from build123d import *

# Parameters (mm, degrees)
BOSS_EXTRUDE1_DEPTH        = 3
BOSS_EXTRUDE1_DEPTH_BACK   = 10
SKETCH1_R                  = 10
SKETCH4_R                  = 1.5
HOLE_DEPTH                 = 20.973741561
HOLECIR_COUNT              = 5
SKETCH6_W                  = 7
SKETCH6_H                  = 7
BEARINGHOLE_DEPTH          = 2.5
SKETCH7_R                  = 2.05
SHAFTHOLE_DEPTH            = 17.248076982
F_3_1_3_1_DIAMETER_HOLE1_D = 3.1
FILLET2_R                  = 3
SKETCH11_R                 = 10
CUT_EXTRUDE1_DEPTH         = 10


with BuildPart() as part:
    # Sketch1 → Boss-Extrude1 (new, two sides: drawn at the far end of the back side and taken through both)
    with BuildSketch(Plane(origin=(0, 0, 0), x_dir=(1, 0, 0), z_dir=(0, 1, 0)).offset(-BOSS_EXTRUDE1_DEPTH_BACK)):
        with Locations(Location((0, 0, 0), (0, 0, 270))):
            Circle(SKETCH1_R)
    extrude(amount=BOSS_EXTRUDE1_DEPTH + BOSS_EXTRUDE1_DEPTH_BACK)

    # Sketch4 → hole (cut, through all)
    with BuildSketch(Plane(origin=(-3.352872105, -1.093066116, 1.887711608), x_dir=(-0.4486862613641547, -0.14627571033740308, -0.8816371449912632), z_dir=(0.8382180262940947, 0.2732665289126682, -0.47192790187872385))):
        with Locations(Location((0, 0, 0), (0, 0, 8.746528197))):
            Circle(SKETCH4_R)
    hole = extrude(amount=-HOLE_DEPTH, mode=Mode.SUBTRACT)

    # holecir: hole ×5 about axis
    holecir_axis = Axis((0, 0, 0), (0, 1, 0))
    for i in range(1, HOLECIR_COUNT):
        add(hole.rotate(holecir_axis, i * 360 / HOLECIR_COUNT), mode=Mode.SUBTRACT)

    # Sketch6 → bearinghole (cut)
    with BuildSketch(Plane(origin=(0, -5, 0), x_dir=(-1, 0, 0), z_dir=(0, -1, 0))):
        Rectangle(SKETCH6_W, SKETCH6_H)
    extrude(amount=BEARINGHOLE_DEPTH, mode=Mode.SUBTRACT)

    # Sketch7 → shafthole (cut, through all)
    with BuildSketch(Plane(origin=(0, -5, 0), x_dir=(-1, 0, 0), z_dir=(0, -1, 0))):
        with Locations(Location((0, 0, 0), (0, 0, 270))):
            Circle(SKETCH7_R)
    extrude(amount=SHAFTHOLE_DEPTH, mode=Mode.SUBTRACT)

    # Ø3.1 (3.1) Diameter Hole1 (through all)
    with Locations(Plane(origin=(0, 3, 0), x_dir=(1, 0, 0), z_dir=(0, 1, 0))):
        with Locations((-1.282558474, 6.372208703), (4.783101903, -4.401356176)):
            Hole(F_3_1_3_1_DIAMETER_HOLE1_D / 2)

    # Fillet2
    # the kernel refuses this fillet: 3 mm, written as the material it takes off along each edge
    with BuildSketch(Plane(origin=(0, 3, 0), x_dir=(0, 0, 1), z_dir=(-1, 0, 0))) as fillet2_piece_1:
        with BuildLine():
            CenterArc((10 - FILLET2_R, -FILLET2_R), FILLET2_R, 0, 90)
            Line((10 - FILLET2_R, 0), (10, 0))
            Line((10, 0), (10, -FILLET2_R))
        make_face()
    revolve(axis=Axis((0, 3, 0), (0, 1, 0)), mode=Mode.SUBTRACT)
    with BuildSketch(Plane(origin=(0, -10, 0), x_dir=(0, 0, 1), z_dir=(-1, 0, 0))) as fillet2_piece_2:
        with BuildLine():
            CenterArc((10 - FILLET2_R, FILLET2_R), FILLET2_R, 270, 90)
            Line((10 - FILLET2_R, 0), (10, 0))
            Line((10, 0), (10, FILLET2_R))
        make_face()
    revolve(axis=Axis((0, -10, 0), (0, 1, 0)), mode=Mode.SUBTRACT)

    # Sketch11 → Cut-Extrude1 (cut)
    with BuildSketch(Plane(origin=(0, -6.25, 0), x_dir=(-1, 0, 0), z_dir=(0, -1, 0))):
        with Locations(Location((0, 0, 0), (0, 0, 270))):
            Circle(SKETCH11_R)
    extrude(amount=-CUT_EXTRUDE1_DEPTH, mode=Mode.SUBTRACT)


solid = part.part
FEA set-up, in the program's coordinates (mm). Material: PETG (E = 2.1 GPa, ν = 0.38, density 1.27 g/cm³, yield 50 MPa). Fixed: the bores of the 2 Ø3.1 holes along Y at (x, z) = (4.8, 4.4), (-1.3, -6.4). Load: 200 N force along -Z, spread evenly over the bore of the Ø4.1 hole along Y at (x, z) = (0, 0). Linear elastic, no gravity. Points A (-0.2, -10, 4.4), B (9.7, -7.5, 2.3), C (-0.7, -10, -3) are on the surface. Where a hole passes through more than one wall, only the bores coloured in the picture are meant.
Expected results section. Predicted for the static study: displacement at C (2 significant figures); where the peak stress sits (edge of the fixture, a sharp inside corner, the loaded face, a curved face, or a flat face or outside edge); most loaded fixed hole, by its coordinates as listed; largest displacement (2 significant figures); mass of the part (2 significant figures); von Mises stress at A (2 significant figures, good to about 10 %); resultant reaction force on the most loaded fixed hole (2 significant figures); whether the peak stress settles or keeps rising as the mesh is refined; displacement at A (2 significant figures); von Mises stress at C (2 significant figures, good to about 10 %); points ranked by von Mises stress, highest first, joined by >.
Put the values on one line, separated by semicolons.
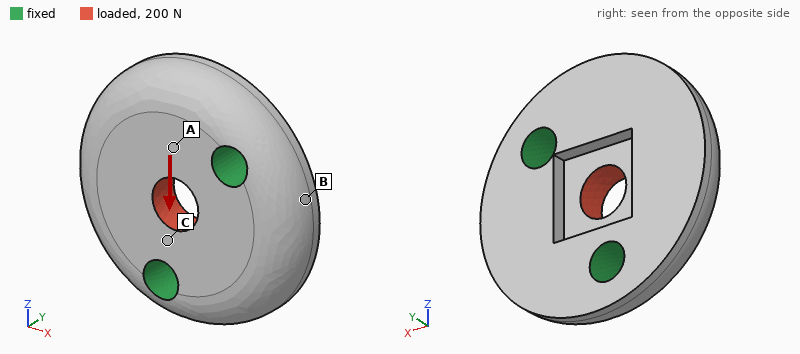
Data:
8.3 µm; edge of the fixture; (-1.3, -6.4); 24 µm; 1.2 g; 4.0 MPa; 110 N; keeps rising; 17 µm; 7.8 MPa; C > A > B
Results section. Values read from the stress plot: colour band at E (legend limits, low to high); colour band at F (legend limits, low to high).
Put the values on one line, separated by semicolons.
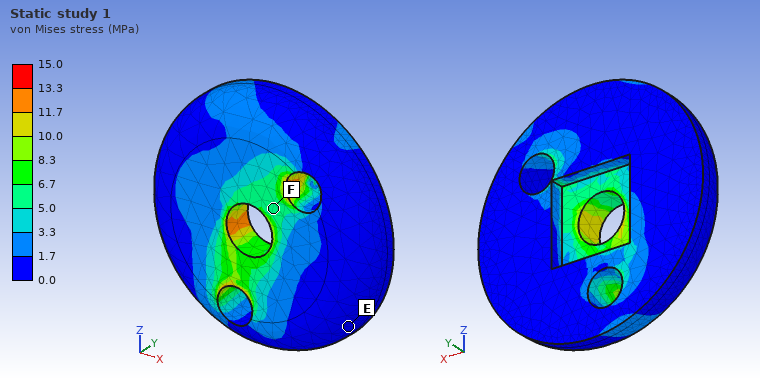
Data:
0.0 to 1.7 MPa; 5.0 to 6.7 MPa
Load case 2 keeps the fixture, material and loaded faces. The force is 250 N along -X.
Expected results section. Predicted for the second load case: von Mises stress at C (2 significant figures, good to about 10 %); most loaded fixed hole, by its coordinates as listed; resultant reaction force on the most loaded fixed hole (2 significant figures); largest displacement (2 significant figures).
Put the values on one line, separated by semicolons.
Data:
5.7 MPa; (4.8, 4.4); 140 N; 31 µm
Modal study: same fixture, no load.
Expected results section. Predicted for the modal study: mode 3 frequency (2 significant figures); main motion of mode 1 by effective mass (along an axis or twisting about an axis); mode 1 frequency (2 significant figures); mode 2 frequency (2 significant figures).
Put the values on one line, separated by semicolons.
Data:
14 kHz; along Y; 6300 Hz; 13 kHz
